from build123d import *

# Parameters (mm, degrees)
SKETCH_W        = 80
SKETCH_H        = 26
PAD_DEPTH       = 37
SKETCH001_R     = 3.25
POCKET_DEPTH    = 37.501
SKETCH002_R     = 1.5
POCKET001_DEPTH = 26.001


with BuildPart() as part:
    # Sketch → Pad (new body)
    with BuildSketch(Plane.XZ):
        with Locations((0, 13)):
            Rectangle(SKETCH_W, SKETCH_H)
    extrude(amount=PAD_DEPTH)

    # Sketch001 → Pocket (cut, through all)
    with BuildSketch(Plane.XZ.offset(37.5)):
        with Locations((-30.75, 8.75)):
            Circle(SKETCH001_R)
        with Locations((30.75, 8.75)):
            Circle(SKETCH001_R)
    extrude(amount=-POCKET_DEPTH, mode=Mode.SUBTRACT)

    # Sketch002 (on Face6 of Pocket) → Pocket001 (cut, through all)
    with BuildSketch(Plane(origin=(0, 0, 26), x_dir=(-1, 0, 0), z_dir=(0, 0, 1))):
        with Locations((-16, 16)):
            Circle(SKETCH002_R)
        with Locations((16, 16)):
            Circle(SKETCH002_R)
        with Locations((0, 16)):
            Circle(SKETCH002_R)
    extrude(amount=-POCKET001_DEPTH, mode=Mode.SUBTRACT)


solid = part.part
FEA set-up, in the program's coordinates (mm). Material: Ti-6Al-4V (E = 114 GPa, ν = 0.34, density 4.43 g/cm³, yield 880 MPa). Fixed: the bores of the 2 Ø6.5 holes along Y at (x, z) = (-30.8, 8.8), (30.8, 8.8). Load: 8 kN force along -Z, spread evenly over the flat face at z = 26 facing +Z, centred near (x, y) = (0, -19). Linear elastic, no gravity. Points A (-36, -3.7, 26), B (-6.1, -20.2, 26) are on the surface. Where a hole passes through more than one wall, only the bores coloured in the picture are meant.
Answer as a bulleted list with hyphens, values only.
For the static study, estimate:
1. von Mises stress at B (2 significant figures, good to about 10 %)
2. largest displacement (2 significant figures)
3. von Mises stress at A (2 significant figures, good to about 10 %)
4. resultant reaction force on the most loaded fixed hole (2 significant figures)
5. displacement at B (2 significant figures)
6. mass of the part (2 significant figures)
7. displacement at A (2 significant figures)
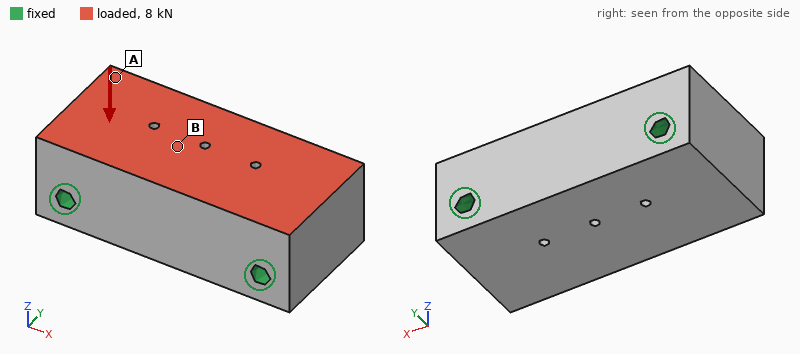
- 6.2 MPa
- 2.8 µm
- 3.0 MPa
- 4.2 kN
- 2.4 µm
- 330 g
- 0.75 µm
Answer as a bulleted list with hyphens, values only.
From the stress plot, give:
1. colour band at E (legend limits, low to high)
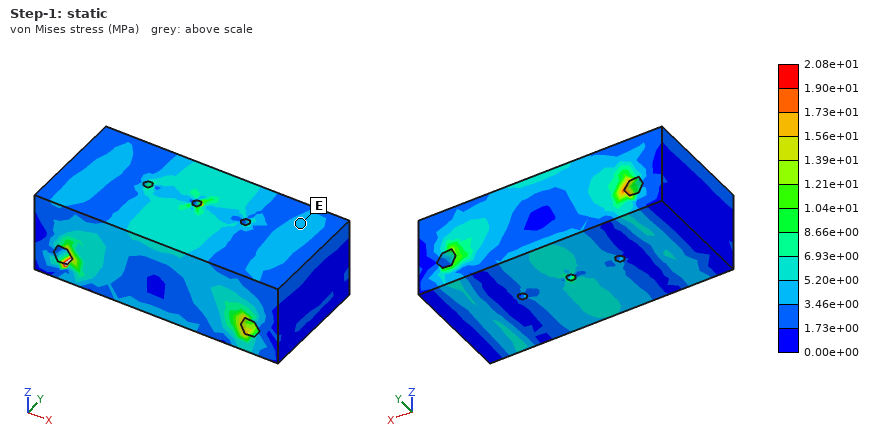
- 3.46e+00 to 5.20e+00 MPa
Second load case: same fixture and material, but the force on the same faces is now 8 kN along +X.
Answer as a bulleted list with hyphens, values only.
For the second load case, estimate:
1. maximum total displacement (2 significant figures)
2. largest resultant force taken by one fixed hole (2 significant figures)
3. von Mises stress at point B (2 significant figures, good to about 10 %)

- 2.6 µm
- 4.4 kN
- 4.7 MPa
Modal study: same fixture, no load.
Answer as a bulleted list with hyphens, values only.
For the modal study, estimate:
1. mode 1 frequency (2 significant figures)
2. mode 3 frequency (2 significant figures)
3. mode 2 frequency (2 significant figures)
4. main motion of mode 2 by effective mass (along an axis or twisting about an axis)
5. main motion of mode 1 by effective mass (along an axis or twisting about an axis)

- 16 kHz
- 22 kHz
- 20 kHz
- along Y
- along Z
